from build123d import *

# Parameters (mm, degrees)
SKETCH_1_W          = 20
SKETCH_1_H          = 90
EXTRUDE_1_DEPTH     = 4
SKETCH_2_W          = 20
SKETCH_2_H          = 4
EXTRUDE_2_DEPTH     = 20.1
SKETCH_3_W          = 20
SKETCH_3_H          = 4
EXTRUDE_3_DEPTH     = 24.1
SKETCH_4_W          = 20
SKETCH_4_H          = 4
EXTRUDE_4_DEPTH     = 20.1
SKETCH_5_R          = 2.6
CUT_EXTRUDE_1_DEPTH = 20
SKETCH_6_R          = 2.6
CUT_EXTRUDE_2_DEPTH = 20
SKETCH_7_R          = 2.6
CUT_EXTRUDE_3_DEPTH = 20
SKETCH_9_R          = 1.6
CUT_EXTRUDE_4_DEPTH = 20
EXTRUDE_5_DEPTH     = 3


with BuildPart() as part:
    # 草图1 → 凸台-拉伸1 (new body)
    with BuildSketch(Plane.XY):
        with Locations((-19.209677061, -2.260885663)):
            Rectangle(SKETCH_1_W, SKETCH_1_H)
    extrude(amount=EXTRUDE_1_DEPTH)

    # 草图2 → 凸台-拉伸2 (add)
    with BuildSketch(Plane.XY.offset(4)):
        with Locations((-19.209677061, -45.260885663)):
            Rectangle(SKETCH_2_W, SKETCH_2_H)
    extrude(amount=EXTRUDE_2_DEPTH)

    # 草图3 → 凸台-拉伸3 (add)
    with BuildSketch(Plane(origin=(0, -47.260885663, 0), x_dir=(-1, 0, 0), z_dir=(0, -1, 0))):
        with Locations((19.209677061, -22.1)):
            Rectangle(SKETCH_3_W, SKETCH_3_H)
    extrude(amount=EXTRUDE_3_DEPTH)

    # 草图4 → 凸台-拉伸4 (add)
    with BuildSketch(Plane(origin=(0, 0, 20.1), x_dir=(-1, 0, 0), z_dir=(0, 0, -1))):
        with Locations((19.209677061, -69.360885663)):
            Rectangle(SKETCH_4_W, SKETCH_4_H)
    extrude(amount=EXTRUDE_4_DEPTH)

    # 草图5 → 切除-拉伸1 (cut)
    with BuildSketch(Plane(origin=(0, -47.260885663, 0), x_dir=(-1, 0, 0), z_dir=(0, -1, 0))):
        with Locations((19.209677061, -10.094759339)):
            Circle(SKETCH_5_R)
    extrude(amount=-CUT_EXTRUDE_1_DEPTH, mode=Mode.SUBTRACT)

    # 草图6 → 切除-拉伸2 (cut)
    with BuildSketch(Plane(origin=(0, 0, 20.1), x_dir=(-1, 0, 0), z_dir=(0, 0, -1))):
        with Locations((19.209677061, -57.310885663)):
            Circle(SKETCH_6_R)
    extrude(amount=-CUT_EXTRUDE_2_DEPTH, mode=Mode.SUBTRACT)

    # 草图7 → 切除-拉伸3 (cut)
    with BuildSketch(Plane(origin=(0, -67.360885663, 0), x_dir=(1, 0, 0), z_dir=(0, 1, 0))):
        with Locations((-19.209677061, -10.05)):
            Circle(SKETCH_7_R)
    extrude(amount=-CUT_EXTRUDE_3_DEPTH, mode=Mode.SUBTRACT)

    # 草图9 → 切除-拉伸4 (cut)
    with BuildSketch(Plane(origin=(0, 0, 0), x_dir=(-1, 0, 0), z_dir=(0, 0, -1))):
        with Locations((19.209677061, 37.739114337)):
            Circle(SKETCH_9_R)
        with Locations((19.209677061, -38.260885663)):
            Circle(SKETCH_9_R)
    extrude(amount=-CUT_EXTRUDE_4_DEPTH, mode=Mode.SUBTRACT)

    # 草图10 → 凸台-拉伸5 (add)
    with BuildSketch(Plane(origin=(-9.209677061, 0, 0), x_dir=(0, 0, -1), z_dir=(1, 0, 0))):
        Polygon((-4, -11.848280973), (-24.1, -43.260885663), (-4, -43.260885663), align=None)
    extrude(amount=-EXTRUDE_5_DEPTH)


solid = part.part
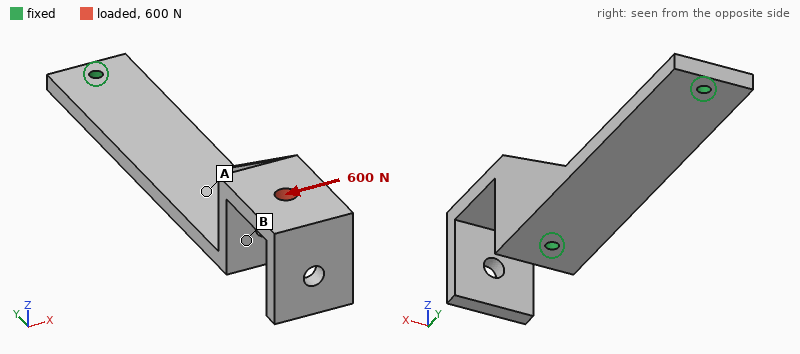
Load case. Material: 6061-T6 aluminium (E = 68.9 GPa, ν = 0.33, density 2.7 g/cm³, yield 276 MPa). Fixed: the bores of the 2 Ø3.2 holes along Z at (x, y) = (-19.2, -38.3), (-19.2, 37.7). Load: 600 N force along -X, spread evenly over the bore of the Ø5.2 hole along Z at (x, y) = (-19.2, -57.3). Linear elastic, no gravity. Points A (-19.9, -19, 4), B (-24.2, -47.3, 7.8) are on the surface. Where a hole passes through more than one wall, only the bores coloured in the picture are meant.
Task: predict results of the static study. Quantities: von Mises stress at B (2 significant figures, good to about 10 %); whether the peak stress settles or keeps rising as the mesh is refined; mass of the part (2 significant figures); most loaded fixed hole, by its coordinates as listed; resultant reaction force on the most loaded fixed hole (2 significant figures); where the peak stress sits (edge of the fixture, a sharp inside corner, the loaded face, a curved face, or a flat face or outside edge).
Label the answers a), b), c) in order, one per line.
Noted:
a) 92 MPa
b) keeps rising
c) 35 g
d) (-19.2, -38.3)
e) 720 N
f) edge of the fixture
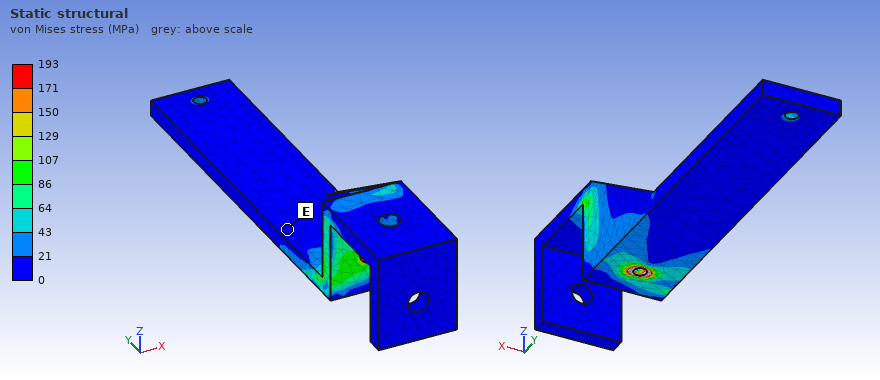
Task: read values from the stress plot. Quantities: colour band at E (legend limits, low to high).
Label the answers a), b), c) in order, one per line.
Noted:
a) 0 to 21 MPa
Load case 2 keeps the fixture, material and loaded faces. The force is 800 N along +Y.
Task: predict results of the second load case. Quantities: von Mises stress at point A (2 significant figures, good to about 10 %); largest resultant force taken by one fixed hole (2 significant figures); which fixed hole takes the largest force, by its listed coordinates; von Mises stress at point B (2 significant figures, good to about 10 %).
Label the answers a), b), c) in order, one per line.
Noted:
a) 33 MPa
b) 630 N
c) (-19.2, -38.3)
d) 93 MPa
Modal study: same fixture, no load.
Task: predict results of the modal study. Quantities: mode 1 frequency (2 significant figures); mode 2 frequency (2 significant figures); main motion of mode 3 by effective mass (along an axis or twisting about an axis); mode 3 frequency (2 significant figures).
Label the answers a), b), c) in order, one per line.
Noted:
a) 1500 Hz
b) 2000 Hz
c) along Y
d) 2800 Hz
